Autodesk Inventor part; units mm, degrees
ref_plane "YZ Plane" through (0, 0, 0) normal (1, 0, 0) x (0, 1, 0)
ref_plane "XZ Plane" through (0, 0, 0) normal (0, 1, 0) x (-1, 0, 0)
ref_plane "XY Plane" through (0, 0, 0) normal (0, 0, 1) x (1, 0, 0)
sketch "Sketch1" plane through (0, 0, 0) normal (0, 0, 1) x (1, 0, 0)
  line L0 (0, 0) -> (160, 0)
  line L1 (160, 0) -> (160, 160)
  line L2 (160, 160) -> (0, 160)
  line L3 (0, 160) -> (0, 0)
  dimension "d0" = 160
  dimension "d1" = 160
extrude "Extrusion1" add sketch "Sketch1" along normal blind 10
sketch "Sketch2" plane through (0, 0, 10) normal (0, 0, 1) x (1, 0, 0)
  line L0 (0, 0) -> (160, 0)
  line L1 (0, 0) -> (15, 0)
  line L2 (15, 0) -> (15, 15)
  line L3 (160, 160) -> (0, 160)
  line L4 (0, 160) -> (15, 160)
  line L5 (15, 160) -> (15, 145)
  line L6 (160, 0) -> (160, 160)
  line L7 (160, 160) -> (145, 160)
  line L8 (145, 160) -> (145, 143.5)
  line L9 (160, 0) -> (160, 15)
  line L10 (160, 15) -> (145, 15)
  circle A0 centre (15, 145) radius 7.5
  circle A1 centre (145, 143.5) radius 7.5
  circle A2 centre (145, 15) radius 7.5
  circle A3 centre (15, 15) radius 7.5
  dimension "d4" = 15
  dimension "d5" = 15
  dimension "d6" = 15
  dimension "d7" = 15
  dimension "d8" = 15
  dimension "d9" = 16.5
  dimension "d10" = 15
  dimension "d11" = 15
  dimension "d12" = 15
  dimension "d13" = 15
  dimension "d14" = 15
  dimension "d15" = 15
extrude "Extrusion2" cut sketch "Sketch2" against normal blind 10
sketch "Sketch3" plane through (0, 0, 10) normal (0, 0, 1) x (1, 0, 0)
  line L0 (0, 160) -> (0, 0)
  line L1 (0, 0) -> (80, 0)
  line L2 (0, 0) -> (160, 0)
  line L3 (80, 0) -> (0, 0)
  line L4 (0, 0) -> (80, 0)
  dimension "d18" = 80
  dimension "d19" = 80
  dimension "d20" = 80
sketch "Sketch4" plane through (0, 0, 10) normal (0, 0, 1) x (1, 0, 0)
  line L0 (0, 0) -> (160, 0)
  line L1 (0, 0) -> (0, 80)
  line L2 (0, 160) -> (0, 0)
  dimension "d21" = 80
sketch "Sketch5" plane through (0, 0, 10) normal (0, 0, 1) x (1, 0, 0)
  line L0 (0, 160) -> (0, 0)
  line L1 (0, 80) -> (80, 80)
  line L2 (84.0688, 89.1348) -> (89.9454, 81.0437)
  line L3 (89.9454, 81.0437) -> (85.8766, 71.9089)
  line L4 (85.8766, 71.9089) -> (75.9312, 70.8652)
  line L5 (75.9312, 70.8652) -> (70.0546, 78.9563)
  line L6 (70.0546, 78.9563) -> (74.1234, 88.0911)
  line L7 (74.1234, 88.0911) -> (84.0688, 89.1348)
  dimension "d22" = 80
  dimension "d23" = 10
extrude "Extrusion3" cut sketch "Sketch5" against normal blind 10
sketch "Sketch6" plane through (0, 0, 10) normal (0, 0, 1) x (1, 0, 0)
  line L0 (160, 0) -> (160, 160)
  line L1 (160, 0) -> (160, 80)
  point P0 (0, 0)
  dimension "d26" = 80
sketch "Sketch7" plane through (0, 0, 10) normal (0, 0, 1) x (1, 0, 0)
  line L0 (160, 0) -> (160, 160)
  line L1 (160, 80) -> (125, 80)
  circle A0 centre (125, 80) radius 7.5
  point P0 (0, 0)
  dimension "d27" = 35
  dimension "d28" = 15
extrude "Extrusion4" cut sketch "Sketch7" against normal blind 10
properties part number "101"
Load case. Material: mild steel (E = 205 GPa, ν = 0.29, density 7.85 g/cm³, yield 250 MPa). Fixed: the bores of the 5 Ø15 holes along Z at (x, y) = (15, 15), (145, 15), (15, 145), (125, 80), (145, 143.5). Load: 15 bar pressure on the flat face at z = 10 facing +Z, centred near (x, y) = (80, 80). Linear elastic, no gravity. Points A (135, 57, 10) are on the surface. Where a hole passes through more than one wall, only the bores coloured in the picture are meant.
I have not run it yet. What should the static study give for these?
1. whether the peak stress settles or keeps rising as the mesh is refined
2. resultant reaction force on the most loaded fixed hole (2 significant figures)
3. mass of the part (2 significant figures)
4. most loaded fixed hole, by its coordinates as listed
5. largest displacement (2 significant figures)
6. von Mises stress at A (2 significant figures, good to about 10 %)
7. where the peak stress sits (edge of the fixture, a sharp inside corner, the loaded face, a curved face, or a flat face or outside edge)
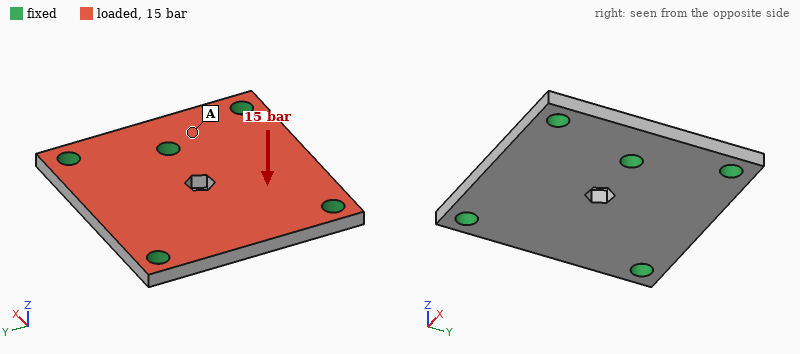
keeps rising
11 kN
1.9 kg
(125, 80)
72 µm
33 MPa
edge of the fixture
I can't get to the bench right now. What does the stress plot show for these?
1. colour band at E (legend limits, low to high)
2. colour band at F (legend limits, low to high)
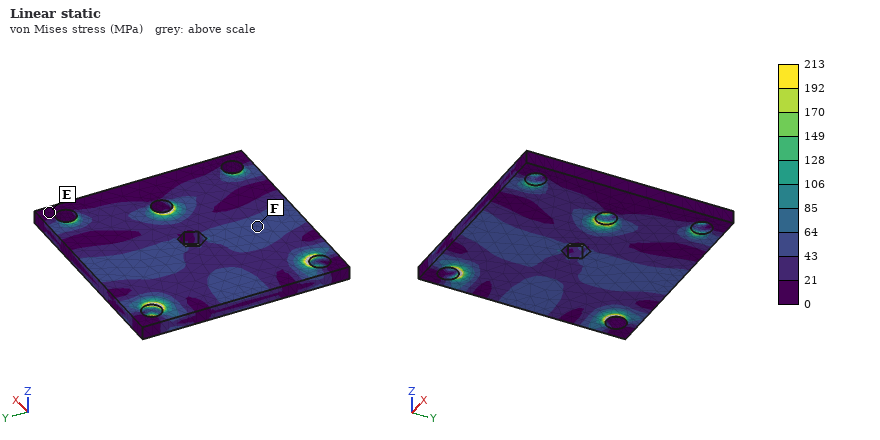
0 to 21 MPa
43 to 64 MPa
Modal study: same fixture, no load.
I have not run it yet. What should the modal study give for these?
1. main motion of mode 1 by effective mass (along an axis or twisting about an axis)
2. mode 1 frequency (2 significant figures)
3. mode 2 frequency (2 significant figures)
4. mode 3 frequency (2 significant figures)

along Z
3100 Hz
3800 Hz
3900 Hz
